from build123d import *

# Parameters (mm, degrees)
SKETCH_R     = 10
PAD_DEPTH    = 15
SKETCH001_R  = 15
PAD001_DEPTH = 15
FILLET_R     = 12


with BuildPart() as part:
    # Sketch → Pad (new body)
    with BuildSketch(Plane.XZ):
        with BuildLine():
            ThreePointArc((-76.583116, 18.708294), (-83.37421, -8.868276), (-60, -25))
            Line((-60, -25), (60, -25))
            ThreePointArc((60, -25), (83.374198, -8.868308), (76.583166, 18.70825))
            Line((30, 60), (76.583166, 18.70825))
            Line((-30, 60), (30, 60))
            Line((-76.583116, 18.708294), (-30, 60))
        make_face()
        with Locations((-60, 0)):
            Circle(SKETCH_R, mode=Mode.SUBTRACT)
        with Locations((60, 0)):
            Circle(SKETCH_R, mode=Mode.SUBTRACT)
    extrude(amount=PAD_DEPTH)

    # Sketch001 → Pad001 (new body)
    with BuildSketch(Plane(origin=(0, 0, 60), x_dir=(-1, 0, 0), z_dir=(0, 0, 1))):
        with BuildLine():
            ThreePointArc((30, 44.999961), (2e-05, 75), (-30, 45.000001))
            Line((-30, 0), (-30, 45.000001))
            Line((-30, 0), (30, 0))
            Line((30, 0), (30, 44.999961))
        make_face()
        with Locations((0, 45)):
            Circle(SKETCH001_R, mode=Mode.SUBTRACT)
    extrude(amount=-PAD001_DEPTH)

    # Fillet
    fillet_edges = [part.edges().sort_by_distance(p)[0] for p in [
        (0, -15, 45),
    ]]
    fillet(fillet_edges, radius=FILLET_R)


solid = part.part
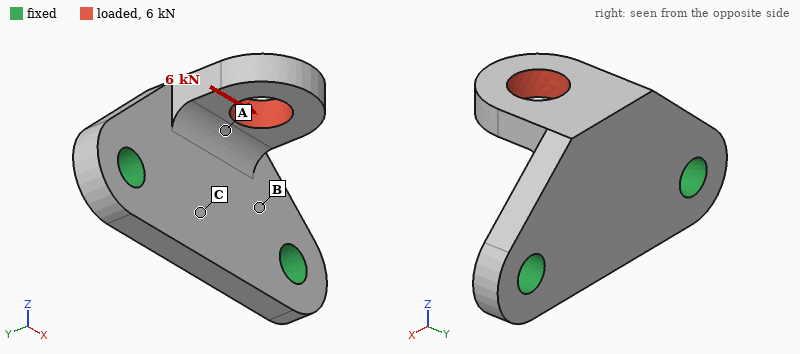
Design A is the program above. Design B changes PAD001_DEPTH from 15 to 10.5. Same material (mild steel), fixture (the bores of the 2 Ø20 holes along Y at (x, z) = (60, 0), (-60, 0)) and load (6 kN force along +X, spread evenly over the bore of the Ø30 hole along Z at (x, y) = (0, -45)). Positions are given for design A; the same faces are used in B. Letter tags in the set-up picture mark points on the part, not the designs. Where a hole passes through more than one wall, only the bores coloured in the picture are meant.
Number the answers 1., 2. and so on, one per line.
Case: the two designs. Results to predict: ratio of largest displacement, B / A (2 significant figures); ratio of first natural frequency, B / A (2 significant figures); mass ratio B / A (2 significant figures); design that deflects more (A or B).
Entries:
1. 1.3
2. 1.0
3. 0.94
4. B
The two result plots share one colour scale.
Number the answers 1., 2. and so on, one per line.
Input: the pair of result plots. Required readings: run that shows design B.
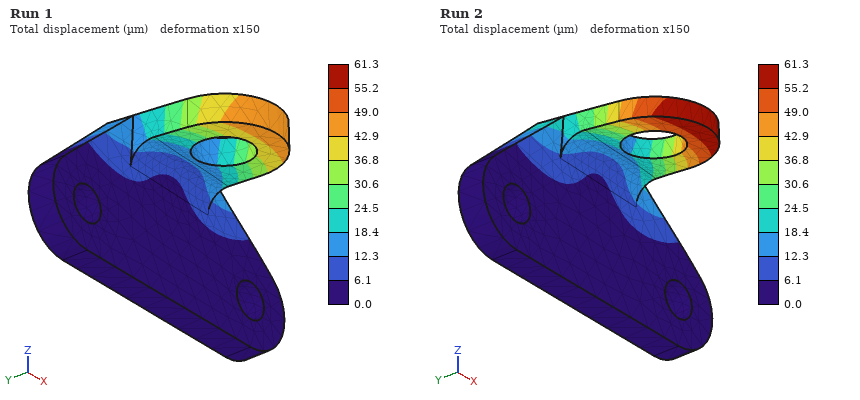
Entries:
1. Run 2
